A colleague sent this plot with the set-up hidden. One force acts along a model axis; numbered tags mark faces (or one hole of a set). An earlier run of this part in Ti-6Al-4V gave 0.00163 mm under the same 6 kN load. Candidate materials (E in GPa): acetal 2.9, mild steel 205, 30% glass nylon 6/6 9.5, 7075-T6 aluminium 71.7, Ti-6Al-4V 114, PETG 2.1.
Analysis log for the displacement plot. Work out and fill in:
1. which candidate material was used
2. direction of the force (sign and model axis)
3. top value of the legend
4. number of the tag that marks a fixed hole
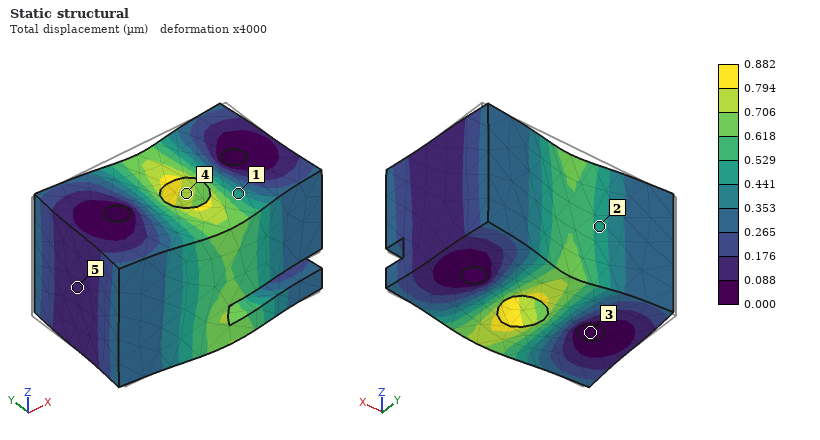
mild steel
-Y
0.882 µm
3
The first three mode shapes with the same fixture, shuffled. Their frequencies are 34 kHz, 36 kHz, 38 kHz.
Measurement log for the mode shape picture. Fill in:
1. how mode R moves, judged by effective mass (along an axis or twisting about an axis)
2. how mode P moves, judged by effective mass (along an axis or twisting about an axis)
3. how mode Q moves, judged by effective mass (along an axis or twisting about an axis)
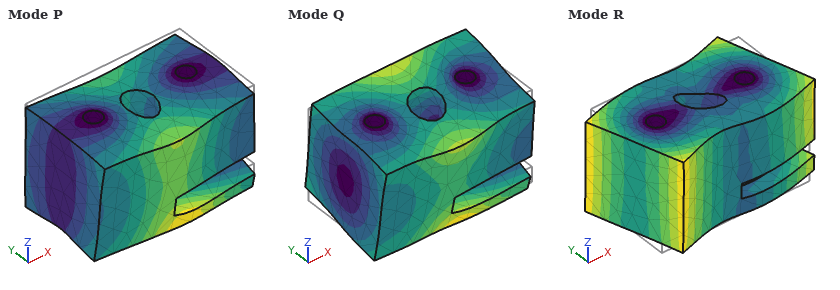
twisting about Z
along Z
twisting about X
